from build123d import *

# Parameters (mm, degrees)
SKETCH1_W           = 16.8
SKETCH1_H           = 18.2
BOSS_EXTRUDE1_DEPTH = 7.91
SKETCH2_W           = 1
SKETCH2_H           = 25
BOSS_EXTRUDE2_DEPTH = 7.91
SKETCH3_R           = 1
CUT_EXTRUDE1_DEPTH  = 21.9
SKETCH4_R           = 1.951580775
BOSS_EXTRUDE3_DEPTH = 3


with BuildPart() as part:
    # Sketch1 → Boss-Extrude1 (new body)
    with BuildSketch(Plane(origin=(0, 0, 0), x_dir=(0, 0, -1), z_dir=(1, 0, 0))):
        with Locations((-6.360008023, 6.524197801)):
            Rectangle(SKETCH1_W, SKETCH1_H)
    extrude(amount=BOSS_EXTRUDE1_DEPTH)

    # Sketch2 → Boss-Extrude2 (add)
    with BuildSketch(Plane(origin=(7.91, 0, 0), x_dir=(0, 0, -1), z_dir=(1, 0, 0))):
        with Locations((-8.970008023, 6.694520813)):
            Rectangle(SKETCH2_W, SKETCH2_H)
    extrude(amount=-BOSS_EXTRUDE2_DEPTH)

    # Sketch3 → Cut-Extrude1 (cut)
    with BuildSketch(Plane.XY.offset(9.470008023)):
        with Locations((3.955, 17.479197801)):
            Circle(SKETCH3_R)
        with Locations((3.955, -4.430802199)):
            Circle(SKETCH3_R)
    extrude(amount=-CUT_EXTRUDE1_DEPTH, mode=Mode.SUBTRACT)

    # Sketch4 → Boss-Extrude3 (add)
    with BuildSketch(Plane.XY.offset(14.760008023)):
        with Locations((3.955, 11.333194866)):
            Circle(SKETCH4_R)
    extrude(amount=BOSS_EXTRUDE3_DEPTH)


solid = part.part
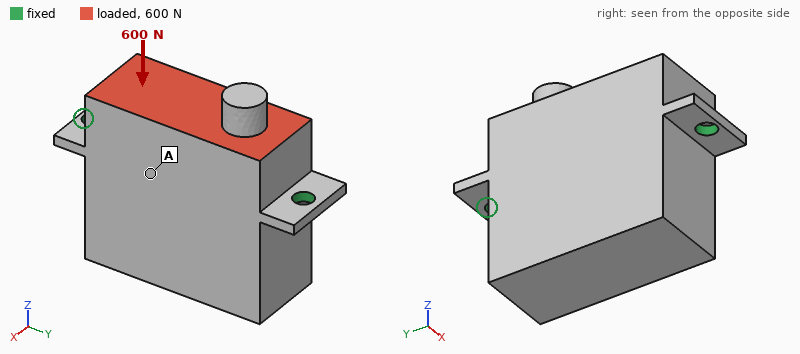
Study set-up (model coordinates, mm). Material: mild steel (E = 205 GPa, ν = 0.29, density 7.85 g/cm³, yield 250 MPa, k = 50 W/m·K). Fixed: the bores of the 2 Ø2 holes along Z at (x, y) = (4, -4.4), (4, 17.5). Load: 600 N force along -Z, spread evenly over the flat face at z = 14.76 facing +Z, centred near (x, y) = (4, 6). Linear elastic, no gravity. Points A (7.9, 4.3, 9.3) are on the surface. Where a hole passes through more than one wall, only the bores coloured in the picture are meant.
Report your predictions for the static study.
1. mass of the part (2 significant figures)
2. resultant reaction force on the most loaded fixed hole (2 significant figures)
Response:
20 g
310 N
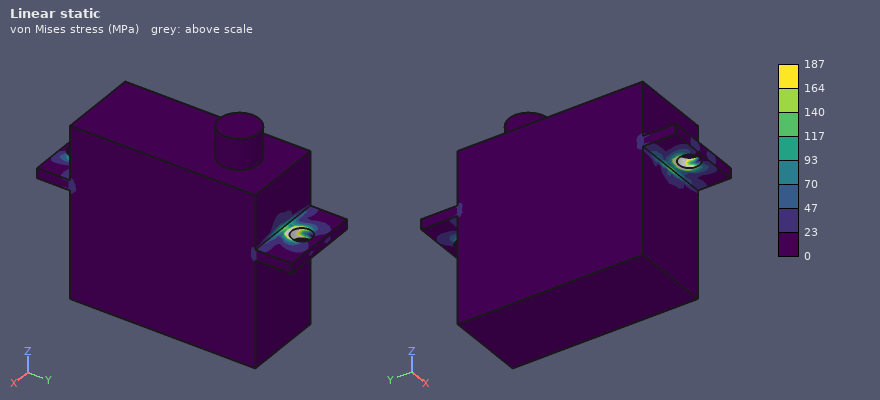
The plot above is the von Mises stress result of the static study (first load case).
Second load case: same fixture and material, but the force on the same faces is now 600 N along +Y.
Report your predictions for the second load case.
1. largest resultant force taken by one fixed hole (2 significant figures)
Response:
350 N
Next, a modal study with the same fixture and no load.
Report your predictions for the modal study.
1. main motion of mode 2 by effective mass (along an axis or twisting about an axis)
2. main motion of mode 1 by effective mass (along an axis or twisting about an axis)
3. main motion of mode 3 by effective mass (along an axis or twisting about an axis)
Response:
along Z
along X
along Y
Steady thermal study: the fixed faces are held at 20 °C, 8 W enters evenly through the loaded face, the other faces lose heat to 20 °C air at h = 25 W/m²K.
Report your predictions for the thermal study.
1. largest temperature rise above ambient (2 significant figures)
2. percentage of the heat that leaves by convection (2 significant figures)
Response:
33 K
8.9 %
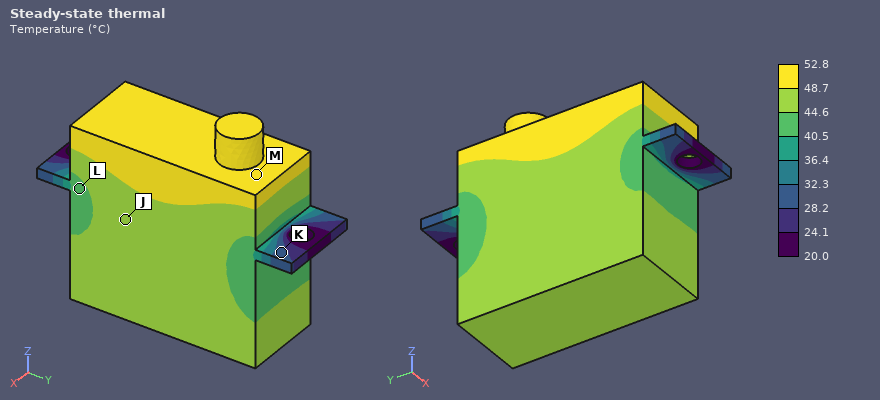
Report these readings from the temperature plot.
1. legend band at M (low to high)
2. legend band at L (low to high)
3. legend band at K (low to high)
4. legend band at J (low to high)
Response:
48.7 to 52.8 °C
40.5 to 44.6 °C
28.2 to 32.3 °C
44.6 to 48.7 °C
